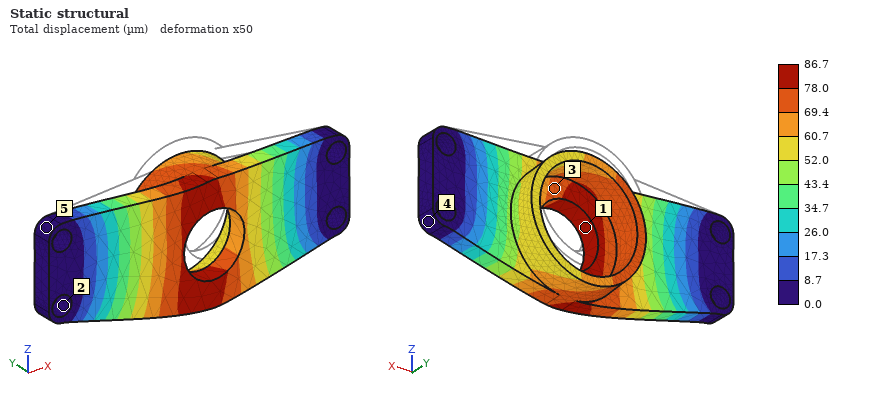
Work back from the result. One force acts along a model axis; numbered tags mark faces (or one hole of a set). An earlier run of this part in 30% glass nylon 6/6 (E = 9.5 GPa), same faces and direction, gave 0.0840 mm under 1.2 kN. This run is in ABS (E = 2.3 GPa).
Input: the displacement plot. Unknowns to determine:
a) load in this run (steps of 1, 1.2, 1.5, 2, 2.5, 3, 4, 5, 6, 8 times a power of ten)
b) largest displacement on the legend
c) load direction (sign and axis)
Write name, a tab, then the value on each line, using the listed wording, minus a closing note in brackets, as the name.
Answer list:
load in this run	300 N
largest displacement on the legend	86.7 µm
load direction	-Z
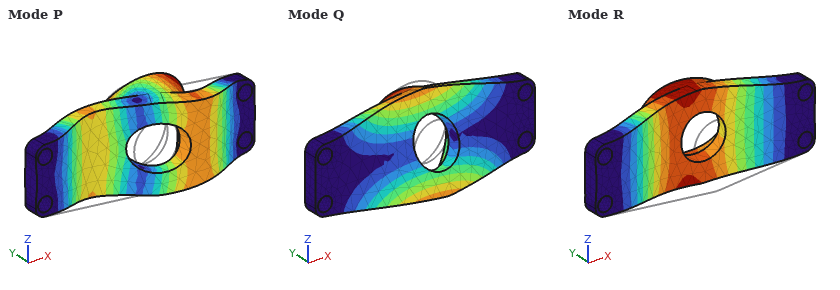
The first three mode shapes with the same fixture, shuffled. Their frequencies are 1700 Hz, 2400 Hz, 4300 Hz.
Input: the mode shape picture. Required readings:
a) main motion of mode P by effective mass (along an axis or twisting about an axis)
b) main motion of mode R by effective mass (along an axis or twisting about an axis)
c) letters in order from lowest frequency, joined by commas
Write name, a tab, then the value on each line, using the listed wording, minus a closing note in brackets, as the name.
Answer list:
main motion of mode P by effective mass	twisting about Z
main motion of mode R by effective mass	along Y
letters in order from lowest frequency, joined by commas	R, Q, P
